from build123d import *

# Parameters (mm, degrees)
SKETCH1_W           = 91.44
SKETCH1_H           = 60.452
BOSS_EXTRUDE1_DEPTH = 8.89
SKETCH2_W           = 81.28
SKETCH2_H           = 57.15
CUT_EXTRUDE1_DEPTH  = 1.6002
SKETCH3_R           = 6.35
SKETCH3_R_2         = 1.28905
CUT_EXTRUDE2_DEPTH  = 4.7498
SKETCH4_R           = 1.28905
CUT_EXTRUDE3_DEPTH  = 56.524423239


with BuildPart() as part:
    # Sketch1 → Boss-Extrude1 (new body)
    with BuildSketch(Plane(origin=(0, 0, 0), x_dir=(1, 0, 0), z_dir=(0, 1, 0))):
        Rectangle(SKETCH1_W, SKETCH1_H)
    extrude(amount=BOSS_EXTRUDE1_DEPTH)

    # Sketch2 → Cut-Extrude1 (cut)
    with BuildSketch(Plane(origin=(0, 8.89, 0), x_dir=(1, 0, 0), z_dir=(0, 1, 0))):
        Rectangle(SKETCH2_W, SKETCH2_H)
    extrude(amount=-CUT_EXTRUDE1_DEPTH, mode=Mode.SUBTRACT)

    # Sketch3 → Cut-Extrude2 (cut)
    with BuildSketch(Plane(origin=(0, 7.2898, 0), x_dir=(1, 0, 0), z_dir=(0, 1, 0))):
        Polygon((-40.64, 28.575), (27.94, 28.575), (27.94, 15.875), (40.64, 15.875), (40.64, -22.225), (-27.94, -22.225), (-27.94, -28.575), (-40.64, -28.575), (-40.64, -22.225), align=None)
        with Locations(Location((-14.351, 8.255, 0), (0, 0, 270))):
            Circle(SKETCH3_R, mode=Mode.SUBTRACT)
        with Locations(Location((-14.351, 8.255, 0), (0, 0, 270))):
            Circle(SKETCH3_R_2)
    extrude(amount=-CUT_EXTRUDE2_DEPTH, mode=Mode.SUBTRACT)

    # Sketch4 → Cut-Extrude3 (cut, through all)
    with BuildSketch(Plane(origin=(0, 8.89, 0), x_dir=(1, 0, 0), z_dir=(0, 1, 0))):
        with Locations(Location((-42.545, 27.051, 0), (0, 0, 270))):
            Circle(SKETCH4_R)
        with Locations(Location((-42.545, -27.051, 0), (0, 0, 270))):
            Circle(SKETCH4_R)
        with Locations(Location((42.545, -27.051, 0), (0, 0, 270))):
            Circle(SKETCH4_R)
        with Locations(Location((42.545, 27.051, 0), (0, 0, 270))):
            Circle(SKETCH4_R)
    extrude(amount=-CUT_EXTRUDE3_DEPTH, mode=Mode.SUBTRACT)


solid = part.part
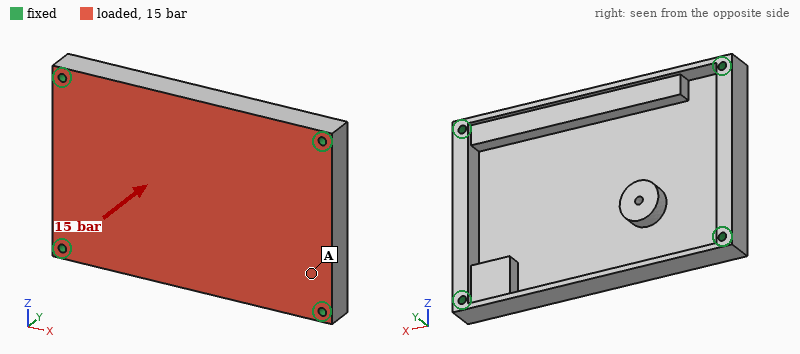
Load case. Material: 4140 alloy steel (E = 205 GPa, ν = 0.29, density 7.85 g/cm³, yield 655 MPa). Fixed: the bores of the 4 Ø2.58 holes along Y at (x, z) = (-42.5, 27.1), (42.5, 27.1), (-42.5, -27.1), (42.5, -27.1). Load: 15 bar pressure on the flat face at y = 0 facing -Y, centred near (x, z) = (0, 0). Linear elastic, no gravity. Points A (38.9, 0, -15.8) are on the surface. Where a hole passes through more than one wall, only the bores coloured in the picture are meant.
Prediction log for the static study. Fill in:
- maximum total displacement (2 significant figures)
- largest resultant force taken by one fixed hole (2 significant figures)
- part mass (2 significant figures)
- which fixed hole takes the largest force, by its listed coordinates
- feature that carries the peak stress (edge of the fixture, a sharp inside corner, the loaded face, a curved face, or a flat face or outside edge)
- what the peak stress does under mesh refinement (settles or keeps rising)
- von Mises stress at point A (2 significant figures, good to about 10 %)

0.26 mm
2.9 kN
180 g
(42.5, -27.1)
edge of the fixture
keeps rising
64 MPa
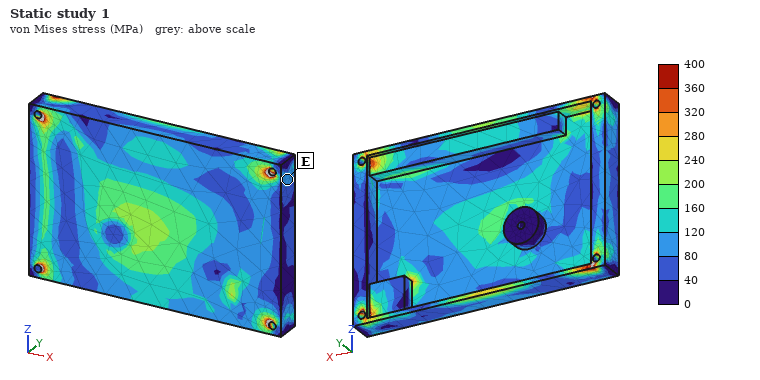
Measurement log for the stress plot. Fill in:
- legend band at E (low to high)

80 to 120 MPa
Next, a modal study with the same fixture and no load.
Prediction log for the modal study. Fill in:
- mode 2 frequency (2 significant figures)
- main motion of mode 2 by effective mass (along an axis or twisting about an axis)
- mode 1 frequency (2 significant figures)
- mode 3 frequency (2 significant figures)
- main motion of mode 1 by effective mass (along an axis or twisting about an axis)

4900 Hz
twisting about X
3100 Hz
6600 Hz
along Y
